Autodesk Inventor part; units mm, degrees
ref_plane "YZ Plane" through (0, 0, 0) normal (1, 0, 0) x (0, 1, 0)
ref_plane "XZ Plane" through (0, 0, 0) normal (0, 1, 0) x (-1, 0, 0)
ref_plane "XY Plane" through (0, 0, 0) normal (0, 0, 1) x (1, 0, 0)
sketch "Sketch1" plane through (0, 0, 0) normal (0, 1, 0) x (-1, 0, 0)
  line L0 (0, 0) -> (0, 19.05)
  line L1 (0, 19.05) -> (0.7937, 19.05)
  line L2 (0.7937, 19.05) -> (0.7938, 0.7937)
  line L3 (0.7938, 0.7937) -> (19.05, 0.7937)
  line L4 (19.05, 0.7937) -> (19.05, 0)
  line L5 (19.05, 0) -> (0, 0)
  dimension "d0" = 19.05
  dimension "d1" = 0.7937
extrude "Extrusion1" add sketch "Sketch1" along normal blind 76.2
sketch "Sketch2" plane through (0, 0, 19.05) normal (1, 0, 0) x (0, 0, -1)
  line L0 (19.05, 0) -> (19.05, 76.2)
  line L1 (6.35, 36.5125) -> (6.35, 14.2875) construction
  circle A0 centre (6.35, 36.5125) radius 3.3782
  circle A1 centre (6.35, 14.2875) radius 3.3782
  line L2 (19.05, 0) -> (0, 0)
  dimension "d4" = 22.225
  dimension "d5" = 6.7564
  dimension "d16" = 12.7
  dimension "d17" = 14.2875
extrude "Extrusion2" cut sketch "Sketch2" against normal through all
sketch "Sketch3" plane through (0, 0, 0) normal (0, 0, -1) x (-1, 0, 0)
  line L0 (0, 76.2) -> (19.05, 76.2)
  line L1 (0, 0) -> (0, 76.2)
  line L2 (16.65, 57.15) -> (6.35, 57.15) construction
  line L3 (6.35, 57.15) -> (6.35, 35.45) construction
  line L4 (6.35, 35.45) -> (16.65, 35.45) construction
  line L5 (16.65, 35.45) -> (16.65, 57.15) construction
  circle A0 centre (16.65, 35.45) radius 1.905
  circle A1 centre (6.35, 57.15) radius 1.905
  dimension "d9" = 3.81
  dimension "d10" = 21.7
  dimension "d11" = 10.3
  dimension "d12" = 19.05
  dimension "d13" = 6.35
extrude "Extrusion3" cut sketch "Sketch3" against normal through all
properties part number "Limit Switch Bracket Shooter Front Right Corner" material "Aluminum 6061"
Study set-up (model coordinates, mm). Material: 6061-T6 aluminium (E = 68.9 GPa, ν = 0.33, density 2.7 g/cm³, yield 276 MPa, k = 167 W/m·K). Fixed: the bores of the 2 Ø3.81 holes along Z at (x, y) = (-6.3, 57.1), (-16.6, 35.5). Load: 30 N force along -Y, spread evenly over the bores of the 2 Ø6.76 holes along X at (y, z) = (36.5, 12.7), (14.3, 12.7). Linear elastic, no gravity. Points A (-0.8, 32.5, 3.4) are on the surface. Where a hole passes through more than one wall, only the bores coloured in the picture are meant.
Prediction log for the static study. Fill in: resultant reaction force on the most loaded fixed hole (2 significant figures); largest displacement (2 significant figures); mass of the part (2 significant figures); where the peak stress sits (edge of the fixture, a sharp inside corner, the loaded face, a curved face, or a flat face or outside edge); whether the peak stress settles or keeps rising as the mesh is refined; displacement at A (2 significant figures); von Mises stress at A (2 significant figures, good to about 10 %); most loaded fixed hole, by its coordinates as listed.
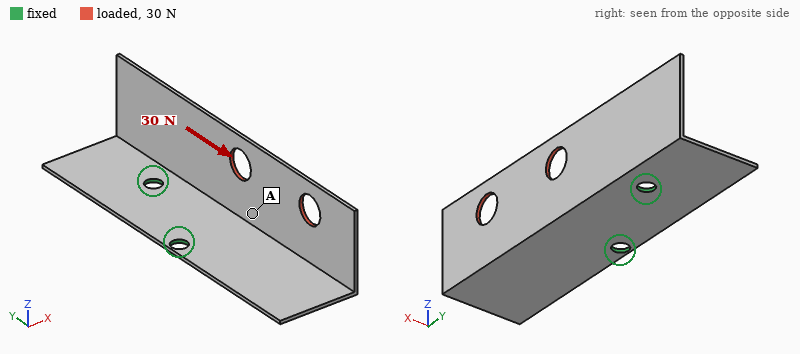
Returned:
28 N
0.37 mm
5.9 g
edge of the fixture
keeps rising
0.13 mm
9.7 MPa
(-6.3, 57.1)
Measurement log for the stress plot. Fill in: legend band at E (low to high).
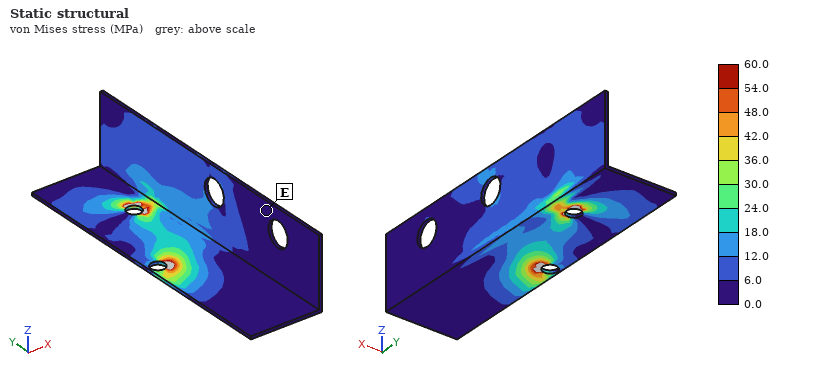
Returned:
0.0 to 6.0 MPa
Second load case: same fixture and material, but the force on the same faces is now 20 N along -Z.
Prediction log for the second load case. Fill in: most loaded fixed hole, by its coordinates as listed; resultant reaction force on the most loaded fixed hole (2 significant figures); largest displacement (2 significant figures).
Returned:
(-16.6, 35.5)
16 N
0.66 mm
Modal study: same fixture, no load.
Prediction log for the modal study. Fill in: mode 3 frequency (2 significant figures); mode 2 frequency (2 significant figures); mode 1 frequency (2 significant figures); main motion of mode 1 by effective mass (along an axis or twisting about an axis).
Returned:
1400 Hz
1000 Hz
630 Hz
along Z
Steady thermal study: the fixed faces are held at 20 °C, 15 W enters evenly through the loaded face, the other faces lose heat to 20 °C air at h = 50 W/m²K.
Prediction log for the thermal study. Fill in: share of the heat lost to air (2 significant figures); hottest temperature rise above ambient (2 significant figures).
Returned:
45 %
68 K
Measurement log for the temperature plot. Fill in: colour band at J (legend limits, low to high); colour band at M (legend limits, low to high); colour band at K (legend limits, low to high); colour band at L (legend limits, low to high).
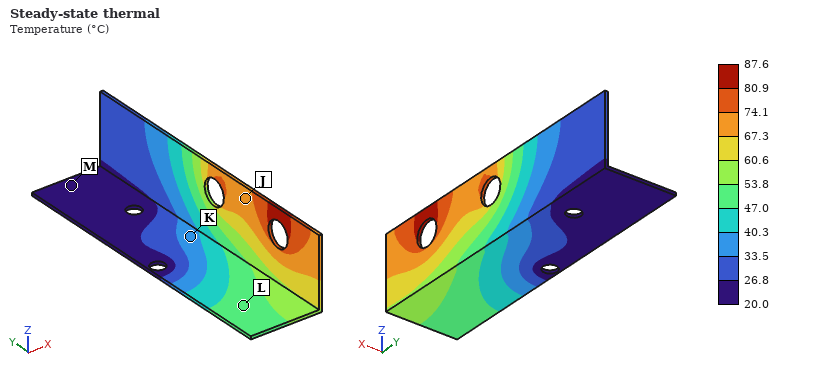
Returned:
67.3 to 74.1 °C
20.0 to 26.8 °C
33.5 to 40.3 °C
47.0 to 53.8 °C
